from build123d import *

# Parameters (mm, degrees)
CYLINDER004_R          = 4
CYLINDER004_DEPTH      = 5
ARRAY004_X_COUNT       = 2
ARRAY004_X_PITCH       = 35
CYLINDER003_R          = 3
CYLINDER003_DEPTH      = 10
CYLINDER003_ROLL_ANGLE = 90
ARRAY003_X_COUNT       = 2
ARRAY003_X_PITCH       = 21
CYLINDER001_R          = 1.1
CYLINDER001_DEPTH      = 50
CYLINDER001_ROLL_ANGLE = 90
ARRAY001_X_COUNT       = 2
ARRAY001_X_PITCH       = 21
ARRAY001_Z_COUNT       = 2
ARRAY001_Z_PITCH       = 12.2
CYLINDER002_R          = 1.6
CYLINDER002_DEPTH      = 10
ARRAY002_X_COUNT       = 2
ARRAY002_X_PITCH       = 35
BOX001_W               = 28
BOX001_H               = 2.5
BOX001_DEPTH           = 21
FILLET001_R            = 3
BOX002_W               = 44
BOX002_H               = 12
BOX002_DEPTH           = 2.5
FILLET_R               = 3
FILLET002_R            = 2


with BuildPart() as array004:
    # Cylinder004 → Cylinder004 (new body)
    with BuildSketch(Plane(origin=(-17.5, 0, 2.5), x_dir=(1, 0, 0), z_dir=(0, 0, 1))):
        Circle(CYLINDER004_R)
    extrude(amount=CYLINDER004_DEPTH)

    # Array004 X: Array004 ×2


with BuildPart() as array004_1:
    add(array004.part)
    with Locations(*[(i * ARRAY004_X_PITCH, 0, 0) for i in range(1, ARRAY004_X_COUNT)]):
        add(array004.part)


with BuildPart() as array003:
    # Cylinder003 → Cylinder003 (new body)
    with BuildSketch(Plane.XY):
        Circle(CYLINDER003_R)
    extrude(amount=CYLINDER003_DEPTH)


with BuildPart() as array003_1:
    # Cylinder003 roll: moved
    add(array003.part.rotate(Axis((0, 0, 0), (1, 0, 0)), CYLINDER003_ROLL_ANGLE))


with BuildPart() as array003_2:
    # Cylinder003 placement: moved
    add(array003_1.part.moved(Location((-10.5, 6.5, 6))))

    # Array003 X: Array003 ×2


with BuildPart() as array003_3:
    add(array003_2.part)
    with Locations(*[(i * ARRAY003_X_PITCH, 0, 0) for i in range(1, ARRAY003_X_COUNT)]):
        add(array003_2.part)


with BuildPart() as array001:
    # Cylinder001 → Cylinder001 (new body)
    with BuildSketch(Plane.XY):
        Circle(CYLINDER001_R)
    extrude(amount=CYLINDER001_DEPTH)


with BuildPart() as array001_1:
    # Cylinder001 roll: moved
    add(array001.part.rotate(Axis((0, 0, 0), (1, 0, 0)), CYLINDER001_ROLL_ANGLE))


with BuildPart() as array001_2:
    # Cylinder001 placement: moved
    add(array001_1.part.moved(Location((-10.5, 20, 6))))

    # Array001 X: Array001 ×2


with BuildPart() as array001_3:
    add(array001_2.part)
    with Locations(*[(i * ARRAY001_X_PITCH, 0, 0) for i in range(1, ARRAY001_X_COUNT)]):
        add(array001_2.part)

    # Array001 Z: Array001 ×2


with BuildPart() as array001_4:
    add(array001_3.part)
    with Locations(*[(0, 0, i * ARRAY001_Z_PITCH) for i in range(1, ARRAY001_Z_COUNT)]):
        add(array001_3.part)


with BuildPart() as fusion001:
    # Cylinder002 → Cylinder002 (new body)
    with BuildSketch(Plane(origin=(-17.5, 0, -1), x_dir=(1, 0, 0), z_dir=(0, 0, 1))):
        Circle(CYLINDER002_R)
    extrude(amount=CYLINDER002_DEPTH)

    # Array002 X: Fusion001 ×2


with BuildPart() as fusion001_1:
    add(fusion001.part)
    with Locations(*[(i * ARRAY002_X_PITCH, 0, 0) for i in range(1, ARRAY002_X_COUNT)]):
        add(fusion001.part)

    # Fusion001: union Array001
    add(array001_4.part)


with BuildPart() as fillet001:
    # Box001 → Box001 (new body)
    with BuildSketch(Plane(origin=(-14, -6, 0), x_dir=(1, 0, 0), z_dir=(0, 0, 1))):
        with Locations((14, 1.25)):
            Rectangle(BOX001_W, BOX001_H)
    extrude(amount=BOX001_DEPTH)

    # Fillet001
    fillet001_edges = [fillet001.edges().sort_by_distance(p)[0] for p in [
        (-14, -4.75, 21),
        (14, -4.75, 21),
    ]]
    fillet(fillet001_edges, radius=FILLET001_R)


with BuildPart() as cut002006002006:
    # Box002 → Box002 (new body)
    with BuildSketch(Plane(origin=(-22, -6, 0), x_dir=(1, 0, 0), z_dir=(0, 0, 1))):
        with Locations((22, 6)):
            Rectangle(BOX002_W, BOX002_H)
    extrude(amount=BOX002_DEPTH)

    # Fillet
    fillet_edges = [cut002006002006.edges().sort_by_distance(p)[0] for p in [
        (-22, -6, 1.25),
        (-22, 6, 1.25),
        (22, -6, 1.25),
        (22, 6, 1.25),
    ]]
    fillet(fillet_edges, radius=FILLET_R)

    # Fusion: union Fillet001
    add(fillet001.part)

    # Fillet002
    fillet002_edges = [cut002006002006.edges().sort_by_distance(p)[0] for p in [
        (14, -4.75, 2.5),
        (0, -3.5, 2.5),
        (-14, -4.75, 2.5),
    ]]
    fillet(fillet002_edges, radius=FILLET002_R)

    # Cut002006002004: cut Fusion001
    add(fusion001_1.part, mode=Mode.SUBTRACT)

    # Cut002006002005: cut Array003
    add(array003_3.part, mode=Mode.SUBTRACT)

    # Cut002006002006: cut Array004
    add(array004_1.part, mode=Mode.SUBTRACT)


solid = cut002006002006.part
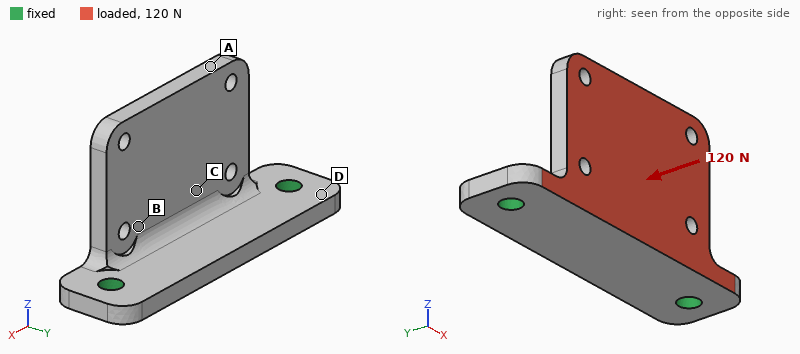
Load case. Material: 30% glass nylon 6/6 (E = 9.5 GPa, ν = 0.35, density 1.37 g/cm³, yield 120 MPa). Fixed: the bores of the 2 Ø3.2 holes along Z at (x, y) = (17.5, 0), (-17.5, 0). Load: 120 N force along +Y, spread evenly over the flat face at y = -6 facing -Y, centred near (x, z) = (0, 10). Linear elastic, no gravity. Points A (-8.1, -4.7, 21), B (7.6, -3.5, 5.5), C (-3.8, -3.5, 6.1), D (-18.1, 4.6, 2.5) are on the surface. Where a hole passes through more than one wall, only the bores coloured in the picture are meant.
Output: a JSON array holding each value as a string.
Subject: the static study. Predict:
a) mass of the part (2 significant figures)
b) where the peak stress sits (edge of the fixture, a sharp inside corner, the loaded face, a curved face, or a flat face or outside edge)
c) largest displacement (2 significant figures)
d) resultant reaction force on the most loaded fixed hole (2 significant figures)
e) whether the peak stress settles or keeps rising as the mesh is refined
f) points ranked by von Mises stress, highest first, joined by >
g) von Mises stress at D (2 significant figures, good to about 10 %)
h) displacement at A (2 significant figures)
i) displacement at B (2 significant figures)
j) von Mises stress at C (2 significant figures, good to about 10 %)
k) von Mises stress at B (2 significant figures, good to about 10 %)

["3.5 g", "edge of the fixture", "0.60 mm", "60 N", "keeps rising", "B > C > D > A", "11 MPa", "0.58 mm", "0.097 mm", "19 MPa", "25 MPa"]
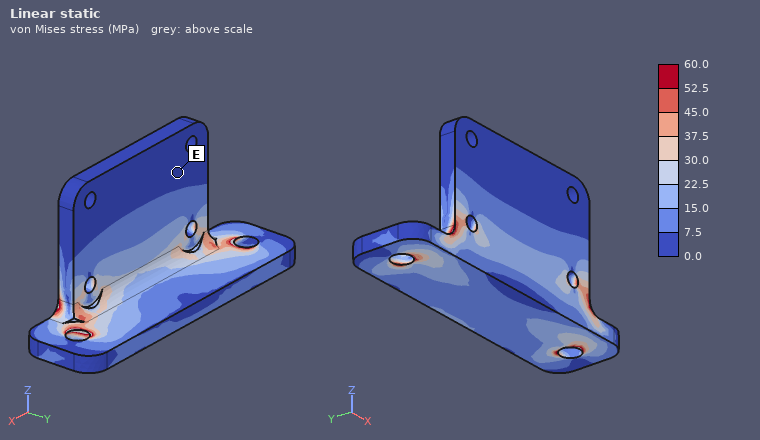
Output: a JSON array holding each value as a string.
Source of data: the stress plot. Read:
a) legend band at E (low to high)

["0.0 to 7.5 MPa"]
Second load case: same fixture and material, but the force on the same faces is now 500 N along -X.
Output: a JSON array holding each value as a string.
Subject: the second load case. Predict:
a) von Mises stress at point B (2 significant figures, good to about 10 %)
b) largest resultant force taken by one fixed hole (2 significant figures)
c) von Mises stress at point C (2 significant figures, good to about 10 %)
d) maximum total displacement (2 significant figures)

["15 MPa", "300 N", "8.4 MPa", "0.10 mm"]
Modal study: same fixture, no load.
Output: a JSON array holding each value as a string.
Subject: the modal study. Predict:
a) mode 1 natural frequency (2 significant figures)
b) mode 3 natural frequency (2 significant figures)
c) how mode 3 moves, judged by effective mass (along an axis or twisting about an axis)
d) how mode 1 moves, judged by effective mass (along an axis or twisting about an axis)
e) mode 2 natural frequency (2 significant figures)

["2000 Hz", "6900 Hz", "along Z", "along Y", "4900 Hz"]
